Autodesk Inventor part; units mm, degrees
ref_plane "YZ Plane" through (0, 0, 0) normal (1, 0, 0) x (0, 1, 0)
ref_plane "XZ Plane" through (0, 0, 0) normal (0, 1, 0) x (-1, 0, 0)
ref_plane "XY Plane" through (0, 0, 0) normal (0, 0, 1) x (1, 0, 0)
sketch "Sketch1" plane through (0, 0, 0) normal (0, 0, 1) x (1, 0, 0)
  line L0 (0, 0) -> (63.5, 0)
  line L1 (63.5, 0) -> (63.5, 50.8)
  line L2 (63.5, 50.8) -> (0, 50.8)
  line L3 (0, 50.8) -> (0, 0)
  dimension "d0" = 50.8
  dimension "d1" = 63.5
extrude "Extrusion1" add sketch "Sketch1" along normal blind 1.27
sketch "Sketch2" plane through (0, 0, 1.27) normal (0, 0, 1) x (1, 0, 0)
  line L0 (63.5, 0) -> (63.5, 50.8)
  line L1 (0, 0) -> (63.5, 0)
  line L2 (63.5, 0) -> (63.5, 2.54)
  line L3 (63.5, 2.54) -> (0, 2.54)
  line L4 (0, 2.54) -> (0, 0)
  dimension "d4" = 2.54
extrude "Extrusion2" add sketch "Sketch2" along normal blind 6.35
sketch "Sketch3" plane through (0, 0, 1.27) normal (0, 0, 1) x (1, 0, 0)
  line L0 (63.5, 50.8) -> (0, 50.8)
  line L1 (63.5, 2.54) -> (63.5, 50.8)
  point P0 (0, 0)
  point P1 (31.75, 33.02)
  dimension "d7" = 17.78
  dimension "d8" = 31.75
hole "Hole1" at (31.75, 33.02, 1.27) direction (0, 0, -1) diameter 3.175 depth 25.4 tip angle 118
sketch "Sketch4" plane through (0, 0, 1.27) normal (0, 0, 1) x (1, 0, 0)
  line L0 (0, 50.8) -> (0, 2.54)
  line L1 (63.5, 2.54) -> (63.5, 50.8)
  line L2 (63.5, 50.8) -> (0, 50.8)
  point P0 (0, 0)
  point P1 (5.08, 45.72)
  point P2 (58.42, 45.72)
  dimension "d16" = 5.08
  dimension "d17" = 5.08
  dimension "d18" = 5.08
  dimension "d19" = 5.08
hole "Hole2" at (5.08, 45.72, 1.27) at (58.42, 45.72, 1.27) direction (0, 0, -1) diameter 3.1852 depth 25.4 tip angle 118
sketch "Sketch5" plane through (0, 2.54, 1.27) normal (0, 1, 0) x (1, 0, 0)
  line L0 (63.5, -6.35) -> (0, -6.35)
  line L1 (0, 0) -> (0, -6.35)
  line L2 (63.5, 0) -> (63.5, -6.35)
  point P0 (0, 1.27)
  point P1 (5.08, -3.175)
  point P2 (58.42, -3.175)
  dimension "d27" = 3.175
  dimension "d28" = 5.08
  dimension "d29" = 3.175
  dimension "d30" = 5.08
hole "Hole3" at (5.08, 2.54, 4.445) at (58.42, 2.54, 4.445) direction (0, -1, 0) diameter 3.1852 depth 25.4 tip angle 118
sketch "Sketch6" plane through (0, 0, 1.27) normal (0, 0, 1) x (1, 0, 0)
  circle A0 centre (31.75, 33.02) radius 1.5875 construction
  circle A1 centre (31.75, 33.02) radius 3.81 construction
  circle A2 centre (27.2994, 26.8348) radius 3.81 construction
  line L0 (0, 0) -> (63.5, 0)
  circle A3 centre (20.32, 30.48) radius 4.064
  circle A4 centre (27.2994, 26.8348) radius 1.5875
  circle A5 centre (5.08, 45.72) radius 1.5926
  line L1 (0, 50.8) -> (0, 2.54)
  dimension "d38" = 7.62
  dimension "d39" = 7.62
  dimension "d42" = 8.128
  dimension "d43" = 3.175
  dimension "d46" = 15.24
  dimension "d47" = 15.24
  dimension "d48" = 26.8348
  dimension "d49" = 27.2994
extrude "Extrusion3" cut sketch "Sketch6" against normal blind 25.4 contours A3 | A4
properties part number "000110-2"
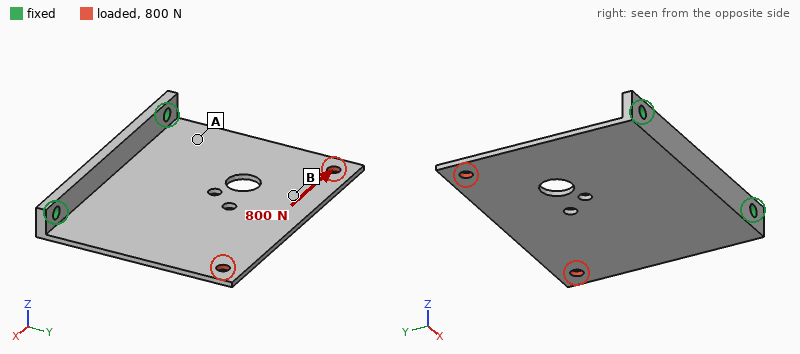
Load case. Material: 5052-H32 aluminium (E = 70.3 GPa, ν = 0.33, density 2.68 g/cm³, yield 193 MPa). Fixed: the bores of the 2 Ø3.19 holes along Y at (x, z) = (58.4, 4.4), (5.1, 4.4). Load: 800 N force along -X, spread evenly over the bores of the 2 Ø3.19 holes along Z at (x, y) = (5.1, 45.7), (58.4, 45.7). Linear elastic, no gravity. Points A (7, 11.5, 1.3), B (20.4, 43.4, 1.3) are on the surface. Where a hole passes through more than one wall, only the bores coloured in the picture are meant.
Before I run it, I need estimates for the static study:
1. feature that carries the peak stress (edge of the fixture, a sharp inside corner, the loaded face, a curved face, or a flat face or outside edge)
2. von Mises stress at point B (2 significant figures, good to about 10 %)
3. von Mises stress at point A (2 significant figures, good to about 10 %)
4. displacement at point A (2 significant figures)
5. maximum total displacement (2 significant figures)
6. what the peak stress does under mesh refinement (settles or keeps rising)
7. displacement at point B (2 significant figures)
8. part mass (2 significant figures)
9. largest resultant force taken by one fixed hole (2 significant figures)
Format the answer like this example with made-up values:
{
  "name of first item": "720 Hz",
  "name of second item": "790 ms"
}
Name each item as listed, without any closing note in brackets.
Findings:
{
  "feature that carries the peak stress": "edge of the fixture",
  "von Mises stress at point B": "24 MPa",
  "von Mises stress at point A": "38 MPa",
  "displacement at point A": "30 µm",
  "maximum total displacement": "98 µm",
  "what the peak stress does under mesh refinement": "keeps rising",
  "displacement at point B": "58 µm",
  "part mass": "13 g",
  "largest resultant force taken by one fixed hole": "780 N"
}
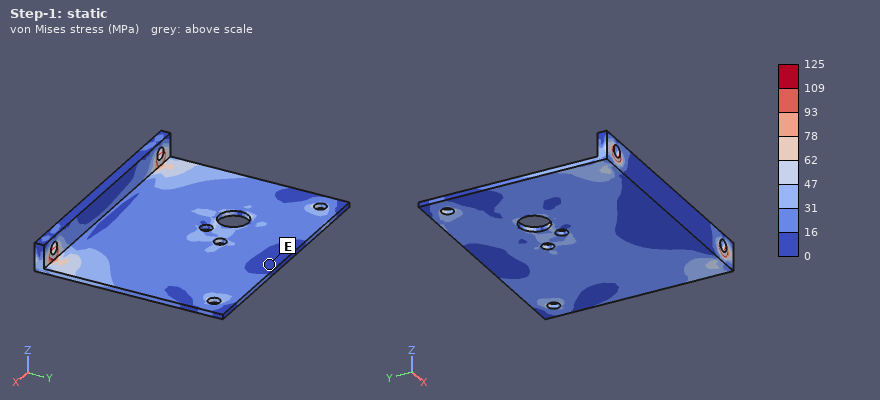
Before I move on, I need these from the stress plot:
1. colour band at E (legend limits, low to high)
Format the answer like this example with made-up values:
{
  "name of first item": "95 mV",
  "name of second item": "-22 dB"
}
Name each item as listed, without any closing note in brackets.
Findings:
{
  "colour band at E": "0 to 16 MPa"
}
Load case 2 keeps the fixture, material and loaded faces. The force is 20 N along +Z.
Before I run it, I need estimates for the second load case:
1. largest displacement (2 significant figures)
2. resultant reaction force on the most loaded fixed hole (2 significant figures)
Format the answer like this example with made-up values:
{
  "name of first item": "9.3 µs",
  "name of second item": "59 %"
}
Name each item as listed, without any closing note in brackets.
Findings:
{
  "largest displacement": "0.96 mm",
  "resultant reaction force on the most loaded fixed hole": "10 N"
}
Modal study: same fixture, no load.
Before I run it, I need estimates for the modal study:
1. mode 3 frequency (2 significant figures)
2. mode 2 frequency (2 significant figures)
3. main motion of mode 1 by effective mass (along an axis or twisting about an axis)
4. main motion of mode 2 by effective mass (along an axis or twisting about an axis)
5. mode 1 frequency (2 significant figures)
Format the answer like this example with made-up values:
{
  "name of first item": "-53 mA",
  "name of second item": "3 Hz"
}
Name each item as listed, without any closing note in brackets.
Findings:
{
  "mode 3 frequency": "2200 Hz",
  "mode 2 frequency": "900 Hz",
  "main motion of mode 1 by effective mass": "along Z",
  "main motion of mode 2 by effective mass": "twisting about Y",
  "mode 1 frequency": "430 Hz"
}
